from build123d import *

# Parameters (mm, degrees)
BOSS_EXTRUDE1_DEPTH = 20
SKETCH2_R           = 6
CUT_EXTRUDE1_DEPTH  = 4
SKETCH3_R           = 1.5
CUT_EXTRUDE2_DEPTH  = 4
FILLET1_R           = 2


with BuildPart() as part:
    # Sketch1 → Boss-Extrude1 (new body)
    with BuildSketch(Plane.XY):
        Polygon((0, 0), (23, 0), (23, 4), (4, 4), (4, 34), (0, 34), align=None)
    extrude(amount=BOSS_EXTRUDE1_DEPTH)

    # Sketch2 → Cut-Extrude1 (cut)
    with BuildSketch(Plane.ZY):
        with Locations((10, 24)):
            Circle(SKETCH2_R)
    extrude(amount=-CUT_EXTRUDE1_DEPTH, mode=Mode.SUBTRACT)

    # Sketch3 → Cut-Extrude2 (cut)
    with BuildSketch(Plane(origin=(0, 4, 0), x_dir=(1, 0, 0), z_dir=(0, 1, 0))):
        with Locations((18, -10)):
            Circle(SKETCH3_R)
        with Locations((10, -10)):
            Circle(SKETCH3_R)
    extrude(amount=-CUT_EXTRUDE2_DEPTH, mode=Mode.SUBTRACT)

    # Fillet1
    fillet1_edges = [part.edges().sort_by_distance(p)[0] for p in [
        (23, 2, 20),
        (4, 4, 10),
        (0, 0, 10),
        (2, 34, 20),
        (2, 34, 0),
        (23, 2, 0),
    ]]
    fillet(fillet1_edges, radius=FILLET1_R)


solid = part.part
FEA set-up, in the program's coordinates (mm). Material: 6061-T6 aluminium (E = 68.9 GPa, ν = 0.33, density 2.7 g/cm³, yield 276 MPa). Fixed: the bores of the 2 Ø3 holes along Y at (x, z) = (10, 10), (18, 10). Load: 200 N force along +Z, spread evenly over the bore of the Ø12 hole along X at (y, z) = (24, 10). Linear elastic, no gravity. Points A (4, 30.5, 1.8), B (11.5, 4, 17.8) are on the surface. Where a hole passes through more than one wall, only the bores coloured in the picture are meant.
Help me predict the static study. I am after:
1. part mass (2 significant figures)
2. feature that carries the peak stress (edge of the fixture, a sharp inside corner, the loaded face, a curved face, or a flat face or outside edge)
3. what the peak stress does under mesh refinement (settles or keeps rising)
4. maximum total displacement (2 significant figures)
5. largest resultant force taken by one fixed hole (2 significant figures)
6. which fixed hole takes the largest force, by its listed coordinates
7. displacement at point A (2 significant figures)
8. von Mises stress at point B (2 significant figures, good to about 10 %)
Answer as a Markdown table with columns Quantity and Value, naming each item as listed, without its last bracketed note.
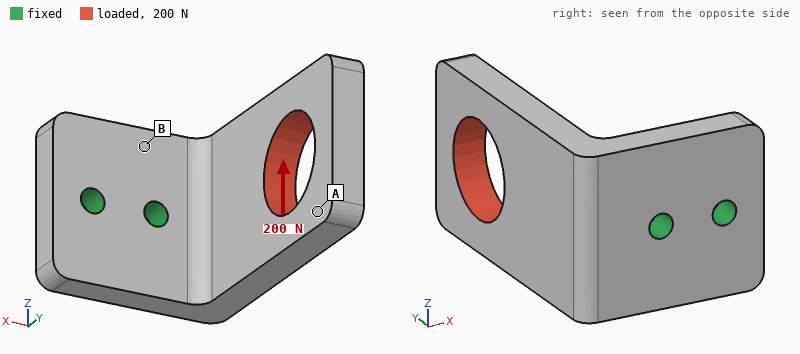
| Quantity | Value |
|---|---|
| part mass | 10 g |
| feature that carries the peak stress | edge of the fixture |
| what the peak stress does under mesh refinement | keeps rising |
| maximum total displacement | 0.11 mm |
| largest resultant force taken by one fixed hole | 320 N |
| which fixed hole takes the largest force, by its listed coordinates | (10, 10) |
| displacement at point A | 0.098 mm |
| von Mises stress at point B | 27 MPa |
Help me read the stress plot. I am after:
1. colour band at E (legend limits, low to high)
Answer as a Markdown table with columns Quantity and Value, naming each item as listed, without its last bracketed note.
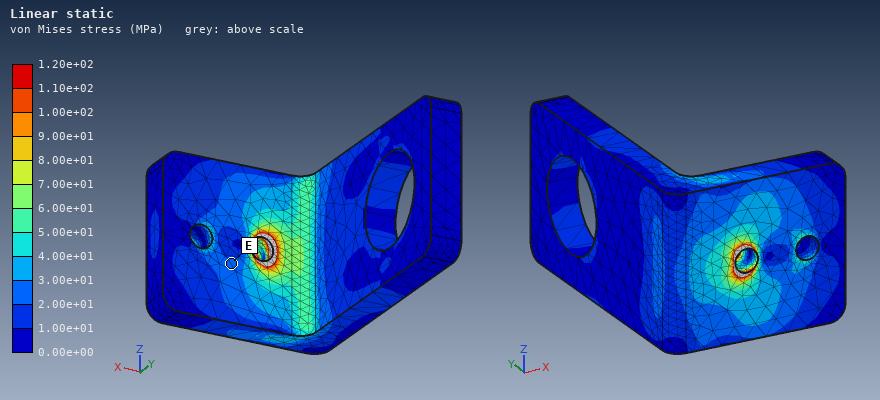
| Quantity | Value |
|---|---|
| colour band at E | 2.00e+01 to 3.00e+01 MPa |
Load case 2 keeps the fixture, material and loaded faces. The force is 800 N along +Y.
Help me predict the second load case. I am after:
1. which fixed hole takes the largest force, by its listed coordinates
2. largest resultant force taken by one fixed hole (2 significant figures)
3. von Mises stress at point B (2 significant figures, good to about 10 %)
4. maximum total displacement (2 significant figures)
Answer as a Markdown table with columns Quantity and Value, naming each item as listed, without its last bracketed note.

| Quantity | Value |
|---|---|
| which fixed hole takes the largest force, by its listed coordinates | (10, 10) |
| largest resultant force taken by one fixed hole | 1.0 kN |
| von Mises stress at point B | 41 MPa |
| maximum total displacement | 0.13 mm |
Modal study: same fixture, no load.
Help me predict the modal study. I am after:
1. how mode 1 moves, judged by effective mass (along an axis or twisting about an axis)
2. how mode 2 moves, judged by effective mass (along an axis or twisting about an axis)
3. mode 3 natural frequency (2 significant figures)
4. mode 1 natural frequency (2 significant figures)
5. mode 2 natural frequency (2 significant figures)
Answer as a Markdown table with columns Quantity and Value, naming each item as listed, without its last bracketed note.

| Quantity | Value |
|---|---|
| how mode 1 moves, judged by effective mass | along X |
| how mode 2 moves, judged by effective mass | along Z |
| mode 3 natural frequency | 9000 Hz |
| mode 1 natural frequency | 2700 Hz |
| mode 2 natural frequency | 4200 Hz |
